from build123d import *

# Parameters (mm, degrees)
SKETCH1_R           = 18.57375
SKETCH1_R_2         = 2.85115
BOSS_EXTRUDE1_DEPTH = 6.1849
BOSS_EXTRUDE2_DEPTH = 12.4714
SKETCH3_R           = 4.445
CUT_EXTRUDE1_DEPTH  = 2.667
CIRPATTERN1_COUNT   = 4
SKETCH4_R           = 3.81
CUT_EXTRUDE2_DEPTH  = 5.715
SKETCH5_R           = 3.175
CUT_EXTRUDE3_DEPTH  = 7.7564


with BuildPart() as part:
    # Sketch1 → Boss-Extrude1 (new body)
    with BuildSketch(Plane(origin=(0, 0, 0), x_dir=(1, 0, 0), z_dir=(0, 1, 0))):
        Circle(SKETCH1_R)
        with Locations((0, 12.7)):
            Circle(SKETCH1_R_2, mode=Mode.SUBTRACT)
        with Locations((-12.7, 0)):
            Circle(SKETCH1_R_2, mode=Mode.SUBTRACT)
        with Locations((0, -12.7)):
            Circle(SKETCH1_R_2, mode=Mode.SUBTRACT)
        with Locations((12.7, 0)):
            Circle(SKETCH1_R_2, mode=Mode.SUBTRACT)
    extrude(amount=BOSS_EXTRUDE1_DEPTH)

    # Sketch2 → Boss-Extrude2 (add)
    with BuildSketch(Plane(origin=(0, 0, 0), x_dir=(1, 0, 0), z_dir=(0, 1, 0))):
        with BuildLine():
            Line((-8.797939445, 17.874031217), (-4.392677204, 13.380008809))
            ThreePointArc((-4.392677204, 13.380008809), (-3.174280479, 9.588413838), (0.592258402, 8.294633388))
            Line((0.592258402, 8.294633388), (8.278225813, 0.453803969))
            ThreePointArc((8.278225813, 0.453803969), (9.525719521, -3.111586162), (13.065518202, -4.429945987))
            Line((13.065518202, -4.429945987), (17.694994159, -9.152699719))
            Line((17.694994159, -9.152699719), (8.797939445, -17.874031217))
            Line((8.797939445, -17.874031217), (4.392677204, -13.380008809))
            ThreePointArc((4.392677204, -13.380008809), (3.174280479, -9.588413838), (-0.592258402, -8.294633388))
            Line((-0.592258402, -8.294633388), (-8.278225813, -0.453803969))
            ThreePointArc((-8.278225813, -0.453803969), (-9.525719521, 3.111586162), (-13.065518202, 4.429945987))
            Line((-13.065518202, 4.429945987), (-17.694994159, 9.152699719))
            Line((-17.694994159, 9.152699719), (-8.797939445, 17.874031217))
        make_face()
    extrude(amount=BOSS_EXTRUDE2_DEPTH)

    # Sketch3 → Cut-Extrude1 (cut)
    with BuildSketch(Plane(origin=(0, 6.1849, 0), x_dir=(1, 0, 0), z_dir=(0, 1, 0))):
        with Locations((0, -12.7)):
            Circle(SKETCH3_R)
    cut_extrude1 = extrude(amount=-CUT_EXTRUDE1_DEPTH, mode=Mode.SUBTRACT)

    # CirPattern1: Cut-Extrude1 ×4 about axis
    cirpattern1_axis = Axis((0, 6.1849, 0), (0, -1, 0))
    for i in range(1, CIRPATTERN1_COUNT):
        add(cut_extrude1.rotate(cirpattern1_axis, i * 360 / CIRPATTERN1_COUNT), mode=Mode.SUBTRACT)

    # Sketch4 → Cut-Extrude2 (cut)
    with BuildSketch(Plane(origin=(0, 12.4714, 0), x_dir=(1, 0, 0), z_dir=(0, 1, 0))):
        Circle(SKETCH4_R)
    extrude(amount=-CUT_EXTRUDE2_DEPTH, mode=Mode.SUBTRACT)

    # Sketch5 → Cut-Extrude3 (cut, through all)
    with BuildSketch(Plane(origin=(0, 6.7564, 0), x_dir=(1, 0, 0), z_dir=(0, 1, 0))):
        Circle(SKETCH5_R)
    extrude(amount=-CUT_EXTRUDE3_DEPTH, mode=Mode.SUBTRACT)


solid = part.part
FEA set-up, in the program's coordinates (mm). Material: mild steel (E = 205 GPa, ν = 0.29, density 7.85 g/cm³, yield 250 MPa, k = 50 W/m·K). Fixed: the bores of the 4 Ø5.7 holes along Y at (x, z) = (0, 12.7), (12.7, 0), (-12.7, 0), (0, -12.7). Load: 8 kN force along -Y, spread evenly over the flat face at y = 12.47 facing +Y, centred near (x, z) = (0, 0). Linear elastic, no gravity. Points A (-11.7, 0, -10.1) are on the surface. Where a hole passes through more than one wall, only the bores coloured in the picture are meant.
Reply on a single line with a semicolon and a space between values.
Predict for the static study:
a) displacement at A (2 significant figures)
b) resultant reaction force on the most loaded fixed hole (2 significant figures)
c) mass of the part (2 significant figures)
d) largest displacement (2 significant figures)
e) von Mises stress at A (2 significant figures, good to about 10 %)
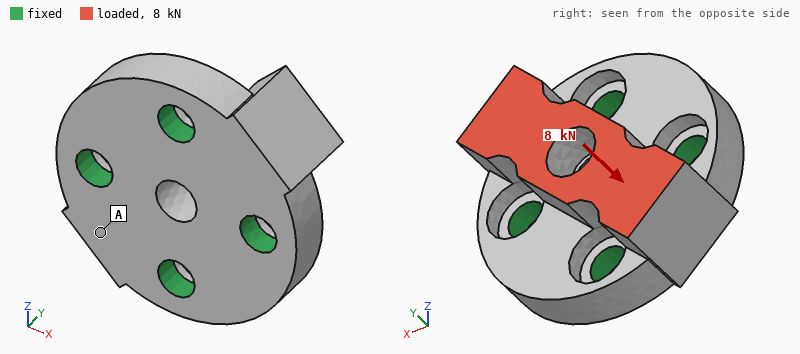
3.8 µm; 2.1 kN; 63 g; 5.3 µm; 24 MPa
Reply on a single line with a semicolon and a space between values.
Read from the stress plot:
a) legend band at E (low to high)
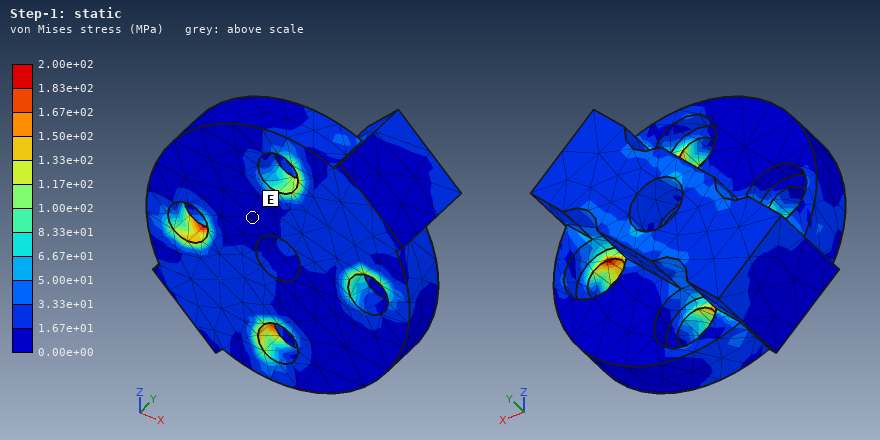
0.00e+00 to 1.67e+01 MPa
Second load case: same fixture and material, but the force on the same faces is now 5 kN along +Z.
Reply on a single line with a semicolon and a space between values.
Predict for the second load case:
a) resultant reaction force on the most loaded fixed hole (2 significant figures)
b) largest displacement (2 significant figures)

2.5 kN; 8.8 µm
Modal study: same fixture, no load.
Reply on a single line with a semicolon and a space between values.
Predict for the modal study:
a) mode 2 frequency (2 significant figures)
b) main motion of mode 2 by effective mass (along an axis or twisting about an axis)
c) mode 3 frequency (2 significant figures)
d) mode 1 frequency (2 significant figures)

36 kHz; along Y; 40 kHz; 29 kHz
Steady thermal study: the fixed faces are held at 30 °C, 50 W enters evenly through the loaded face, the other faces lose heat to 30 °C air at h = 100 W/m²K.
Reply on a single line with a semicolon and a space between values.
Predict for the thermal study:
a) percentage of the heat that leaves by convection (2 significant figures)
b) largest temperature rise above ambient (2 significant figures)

8.7 %; 37 K
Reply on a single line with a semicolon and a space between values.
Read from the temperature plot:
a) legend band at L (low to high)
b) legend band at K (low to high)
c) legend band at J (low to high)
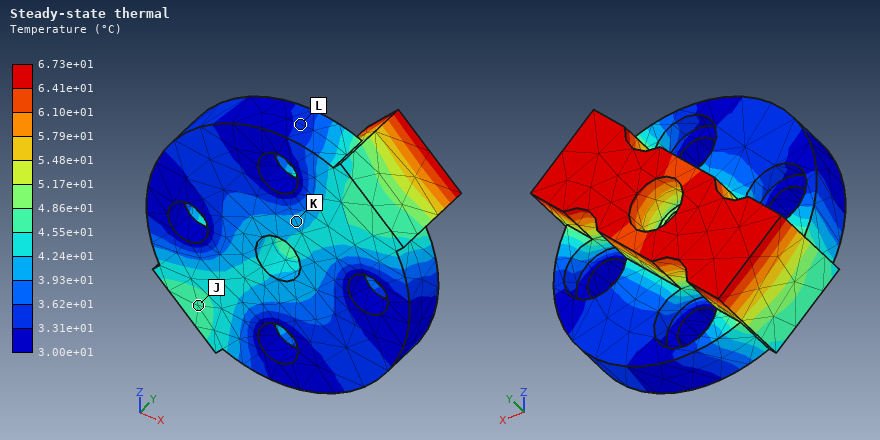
3.31e+01 to 3.62e+01 °C; 3.93e+01 to 4.24e+01 °C; 4.55e+01 to 4.86e+01 °C
